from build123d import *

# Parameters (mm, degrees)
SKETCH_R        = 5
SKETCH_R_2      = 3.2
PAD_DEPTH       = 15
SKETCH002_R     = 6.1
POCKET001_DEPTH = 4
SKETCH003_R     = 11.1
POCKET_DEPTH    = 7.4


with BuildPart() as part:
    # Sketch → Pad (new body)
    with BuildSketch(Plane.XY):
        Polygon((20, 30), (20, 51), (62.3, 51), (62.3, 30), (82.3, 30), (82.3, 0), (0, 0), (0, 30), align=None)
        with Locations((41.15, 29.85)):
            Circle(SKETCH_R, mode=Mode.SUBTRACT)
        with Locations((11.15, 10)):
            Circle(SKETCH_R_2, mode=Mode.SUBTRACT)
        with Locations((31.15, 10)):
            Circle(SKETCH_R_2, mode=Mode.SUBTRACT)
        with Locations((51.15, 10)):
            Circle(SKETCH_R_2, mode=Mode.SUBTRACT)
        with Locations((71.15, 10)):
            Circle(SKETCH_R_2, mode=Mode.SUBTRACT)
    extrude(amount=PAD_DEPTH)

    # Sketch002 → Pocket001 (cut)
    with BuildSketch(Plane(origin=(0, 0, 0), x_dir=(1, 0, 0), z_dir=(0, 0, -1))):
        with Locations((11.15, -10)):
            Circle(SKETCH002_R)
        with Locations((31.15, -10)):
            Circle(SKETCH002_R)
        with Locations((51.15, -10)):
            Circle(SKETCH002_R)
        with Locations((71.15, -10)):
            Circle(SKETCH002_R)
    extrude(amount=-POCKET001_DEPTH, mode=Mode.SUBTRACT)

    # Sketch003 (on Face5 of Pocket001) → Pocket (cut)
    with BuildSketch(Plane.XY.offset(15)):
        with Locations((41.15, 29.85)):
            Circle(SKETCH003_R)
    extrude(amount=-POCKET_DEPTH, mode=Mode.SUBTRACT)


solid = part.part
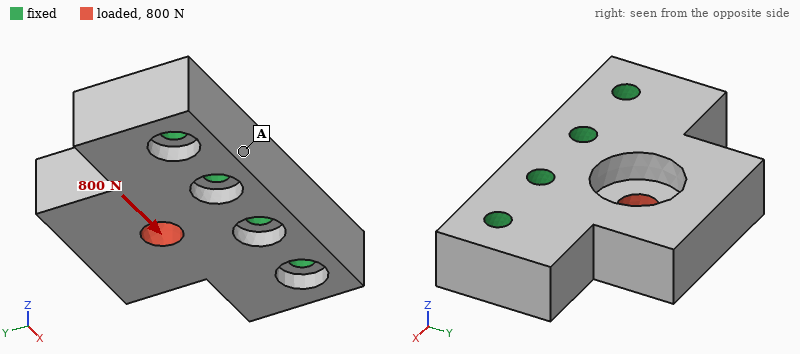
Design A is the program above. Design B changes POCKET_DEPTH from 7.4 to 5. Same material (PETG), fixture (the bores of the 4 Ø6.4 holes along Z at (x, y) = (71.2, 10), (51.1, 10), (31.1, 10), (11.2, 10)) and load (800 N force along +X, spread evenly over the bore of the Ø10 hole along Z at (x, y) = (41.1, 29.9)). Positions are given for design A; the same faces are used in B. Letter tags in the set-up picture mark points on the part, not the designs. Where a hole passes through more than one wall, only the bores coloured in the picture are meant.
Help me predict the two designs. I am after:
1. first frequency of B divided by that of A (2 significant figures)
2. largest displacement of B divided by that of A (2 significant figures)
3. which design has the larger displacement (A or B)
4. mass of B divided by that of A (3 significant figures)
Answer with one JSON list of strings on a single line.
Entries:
["1.0", "0.86", "A", "1.02"]
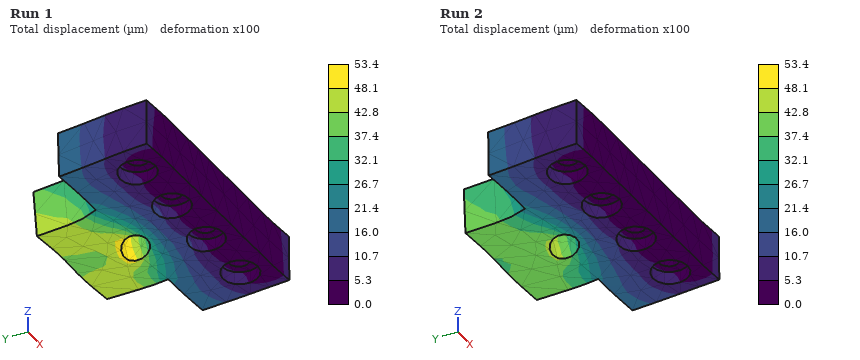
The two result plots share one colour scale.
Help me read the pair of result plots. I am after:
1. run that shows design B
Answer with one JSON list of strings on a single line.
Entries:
["Run 2"]
